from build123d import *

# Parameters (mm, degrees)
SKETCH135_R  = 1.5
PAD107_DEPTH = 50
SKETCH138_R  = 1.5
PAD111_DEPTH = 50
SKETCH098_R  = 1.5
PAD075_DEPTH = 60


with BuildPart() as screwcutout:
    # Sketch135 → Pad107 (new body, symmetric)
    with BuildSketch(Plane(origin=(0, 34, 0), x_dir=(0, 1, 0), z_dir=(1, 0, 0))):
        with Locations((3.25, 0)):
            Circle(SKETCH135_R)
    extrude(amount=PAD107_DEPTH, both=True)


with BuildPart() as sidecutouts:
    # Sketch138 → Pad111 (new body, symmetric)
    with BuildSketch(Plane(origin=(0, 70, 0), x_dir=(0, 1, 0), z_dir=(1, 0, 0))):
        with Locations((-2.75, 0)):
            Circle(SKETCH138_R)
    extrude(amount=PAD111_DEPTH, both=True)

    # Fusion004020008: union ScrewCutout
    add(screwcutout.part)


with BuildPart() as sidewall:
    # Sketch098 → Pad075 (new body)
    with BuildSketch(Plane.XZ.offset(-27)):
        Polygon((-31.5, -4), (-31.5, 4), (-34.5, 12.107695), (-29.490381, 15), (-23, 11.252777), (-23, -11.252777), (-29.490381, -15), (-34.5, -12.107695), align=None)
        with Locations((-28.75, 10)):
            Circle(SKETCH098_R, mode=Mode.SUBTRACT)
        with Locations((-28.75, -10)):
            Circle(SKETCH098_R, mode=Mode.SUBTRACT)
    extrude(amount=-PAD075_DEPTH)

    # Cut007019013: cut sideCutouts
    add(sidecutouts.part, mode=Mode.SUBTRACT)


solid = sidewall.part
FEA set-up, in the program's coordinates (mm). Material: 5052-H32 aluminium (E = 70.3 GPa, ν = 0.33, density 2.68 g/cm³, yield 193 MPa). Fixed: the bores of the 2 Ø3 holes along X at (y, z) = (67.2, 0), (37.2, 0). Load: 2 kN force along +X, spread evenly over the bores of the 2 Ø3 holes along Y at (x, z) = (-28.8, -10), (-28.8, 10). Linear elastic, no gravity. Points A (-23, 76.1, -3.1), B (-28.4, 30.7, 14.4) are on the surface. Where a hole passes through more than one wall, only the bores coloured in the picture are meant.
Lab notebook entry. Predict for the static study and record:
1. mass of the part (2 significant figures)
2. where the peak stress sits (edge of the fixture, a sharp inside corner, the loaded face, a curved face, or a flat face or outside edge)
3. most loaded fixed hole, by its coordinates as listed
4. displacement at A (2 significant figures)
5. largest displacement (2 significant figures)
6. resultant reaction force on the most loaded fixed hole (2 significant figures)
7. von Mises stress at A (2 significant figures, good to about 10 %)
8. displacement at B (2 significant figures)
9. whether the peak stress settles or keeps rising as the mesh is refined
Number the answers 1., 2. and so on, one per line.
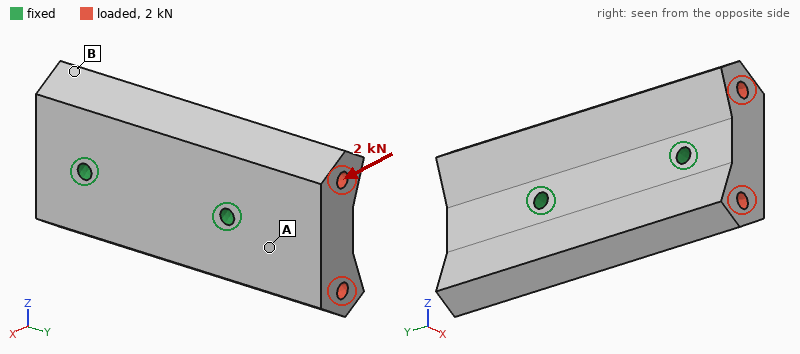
1. 39 g
2. edge of the fixture
3. (67.2, 0)
4. 4.3 µm
5. 10.0 µm
6. 1.2 kN
7. 8.4 MPa
8. 3.4 µm
9. keeps rising
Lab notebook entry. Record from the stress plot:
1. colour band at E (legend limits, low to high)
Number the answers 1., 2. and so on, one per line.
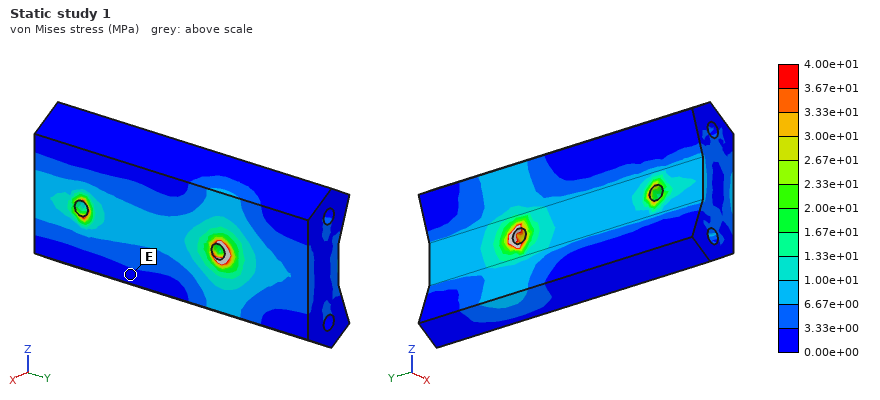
1. 0.00e+00 to 3.33e+00 MPa
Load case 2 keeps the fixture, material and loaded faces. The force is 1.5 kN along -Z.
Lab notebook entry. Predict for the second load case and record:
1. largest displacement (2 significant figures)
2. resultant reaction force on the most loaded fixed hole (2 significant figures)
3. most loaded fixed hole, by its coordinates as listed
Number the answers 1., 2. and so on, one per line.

1. 4.1 µm
2. 970 N
3. (67.2, 0)
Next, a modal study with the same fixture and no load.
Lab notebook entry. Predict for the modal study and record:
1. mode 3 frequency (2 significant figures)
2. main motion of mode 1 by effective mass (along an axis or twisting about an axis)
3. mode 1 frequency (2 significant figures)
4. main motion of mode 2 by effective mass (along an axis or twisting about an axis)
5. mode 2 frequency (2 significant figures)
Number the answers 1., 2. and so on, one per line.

1. 19 kHz
2. along X
3. 13 kHz
4. twisting about Y
5. 15 kHz
